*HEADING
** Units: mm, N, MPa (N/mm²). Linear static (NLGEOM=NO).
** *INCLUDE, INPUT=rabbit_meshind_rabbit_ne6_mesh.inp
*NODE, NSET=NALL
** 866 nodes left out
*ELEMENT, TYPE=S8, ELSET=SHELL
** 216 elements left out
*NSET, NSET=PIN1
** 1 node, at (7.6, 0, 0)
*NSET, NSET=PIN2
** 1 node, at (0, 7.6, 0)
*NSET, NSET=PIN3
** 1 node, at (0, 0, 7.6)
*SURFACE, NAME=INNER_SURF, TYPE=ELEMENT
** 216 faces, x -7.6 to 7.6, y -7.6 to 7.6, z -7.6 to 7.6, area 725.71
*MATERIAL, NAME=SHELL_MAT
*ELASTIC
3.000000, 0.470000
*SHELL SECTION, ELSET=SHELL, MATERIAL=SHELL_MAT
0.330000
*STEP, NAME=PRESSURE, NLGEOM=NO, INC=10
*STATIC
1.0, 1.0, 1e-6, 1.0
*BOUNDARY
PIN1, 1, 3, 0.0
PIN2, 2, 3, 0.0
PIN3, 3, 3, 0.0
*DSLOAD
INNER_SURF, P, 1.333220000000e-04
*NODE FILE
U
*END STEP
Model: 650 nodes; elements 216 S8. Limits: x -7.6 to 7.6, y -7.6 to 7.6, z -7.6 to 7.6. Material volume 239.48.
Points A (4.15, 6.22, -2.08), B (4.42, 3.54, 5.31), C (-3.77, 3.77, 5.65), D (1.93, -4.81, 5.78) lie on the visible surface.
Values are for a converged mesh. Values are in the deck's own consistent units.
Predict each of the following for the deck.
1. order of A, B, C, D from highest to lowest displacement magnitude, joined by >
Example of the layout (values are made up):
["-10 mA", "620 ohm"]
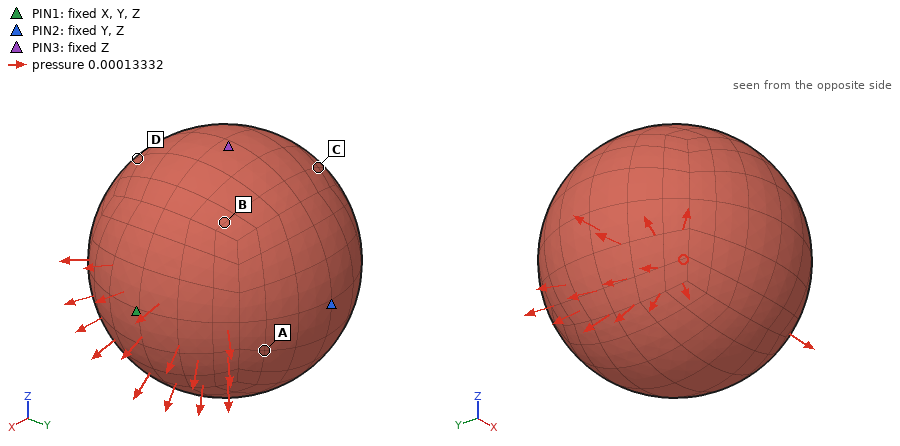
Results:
["C > D > B > A"]
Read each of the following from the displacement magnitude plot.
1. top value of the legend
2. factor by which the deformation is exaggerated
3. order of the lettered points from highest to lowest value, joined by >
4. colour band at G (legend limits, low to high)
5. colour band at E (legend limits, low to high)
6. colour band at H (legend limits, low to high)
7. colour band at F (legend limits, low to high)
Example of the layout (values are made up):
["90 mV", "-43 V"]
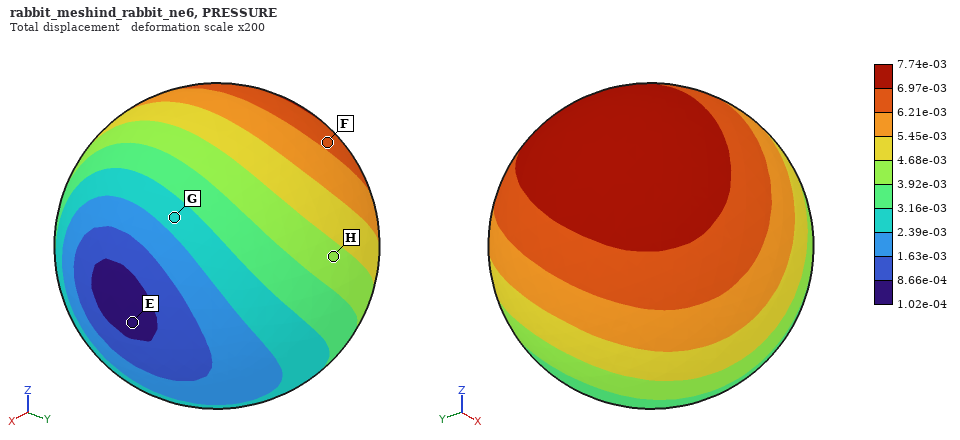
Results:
["7.74e-03", "200", "F > H > G > E", "2.39e-03 to 3.16e-03", "1.02e-04 to 8.66e-04", "3.92e-03 to 4.68e-03", "6.21e-03 to 6.97e-03"]
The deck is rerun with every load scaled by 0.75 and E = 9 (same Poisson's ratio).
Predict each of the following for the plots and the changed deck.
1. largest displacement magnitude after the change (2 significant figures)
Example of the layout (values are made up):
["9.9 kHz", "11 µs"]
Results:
["0.0019"]
